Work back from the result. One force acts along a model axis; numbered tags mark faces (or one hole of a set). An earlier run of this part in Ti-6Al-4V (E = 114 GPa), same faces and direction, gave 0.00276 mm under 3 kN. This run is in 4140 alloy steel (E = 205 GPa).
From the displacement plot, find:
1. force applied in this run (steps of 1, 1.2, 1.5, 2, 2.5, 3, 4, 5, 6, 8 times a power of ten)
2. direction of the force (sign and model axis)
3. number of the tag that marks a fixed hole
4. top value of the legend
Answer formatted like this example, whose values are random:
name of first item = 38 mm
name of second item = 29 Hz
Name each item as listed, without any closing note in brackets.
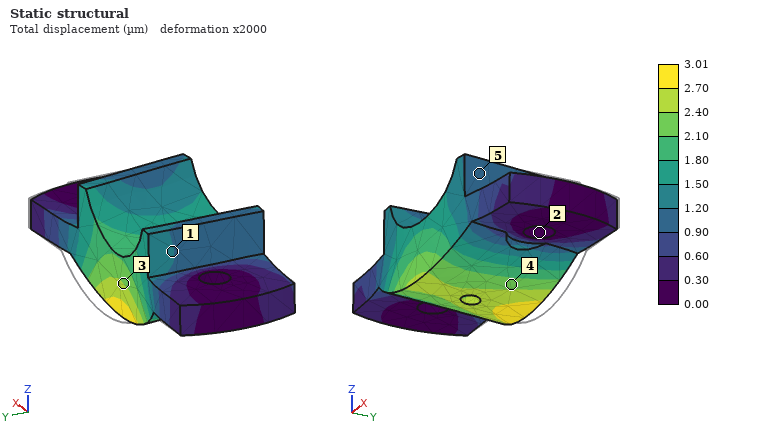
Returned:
force applied in this run = 6 kN
direction of the force = -Y
number of the tag that marks a fixed hole = 2
top value of the legend = 3.01 µm
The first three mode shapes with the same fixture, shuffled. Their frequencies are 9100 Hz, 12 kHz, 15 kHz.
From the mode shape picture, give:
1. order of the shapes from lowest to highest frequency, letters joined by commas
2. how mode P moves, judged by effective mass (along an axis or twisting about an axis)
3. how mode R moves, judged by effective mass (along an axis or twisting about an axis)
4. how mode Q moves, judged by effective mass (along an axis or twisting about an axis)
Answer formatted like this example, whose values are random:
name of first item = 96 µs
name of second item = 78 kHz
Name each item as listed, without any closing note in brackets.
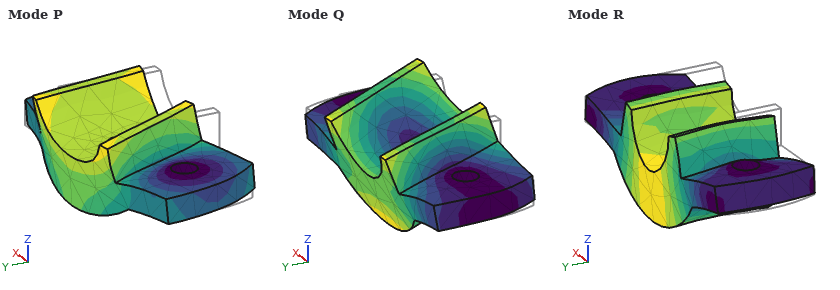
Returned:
order of the shapes from lowest to highest frequency, letters joined by commas = Q, R, P
how mode P moves, judged by effective mass = along Y
how mode R moves, judged by effective mass = along Z
how mode Q moves, judged by effective mass = twisting about X
